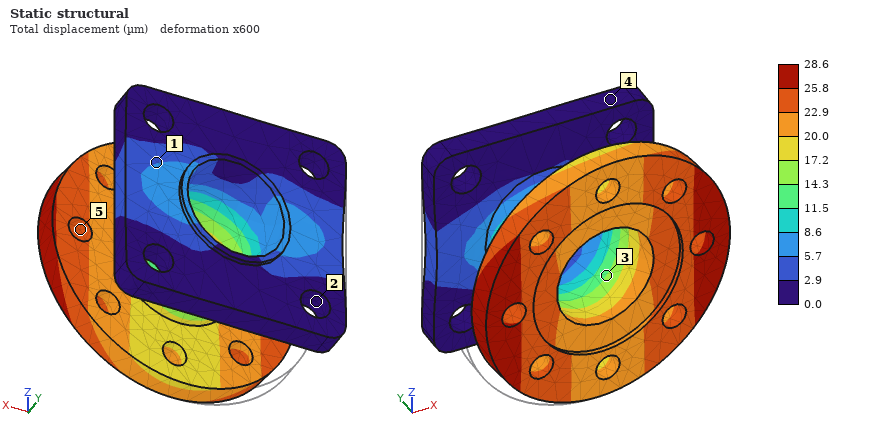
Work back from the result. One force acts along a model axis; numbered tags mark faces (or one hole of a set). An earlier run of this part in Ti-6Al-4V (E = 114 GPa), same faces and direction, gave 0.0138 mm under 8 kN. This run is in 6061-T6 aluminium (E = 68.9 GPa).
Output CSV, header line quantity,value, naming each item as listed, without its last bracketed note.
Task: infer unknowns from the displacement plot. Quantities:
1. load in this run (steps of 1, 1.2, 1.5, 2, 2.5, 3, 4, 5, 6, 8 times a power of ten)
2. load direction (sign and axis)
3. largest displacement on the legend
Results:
quantity,value
load in this run,10 kN
load direction,+X
largest displacement on the legend,28.6 µm
